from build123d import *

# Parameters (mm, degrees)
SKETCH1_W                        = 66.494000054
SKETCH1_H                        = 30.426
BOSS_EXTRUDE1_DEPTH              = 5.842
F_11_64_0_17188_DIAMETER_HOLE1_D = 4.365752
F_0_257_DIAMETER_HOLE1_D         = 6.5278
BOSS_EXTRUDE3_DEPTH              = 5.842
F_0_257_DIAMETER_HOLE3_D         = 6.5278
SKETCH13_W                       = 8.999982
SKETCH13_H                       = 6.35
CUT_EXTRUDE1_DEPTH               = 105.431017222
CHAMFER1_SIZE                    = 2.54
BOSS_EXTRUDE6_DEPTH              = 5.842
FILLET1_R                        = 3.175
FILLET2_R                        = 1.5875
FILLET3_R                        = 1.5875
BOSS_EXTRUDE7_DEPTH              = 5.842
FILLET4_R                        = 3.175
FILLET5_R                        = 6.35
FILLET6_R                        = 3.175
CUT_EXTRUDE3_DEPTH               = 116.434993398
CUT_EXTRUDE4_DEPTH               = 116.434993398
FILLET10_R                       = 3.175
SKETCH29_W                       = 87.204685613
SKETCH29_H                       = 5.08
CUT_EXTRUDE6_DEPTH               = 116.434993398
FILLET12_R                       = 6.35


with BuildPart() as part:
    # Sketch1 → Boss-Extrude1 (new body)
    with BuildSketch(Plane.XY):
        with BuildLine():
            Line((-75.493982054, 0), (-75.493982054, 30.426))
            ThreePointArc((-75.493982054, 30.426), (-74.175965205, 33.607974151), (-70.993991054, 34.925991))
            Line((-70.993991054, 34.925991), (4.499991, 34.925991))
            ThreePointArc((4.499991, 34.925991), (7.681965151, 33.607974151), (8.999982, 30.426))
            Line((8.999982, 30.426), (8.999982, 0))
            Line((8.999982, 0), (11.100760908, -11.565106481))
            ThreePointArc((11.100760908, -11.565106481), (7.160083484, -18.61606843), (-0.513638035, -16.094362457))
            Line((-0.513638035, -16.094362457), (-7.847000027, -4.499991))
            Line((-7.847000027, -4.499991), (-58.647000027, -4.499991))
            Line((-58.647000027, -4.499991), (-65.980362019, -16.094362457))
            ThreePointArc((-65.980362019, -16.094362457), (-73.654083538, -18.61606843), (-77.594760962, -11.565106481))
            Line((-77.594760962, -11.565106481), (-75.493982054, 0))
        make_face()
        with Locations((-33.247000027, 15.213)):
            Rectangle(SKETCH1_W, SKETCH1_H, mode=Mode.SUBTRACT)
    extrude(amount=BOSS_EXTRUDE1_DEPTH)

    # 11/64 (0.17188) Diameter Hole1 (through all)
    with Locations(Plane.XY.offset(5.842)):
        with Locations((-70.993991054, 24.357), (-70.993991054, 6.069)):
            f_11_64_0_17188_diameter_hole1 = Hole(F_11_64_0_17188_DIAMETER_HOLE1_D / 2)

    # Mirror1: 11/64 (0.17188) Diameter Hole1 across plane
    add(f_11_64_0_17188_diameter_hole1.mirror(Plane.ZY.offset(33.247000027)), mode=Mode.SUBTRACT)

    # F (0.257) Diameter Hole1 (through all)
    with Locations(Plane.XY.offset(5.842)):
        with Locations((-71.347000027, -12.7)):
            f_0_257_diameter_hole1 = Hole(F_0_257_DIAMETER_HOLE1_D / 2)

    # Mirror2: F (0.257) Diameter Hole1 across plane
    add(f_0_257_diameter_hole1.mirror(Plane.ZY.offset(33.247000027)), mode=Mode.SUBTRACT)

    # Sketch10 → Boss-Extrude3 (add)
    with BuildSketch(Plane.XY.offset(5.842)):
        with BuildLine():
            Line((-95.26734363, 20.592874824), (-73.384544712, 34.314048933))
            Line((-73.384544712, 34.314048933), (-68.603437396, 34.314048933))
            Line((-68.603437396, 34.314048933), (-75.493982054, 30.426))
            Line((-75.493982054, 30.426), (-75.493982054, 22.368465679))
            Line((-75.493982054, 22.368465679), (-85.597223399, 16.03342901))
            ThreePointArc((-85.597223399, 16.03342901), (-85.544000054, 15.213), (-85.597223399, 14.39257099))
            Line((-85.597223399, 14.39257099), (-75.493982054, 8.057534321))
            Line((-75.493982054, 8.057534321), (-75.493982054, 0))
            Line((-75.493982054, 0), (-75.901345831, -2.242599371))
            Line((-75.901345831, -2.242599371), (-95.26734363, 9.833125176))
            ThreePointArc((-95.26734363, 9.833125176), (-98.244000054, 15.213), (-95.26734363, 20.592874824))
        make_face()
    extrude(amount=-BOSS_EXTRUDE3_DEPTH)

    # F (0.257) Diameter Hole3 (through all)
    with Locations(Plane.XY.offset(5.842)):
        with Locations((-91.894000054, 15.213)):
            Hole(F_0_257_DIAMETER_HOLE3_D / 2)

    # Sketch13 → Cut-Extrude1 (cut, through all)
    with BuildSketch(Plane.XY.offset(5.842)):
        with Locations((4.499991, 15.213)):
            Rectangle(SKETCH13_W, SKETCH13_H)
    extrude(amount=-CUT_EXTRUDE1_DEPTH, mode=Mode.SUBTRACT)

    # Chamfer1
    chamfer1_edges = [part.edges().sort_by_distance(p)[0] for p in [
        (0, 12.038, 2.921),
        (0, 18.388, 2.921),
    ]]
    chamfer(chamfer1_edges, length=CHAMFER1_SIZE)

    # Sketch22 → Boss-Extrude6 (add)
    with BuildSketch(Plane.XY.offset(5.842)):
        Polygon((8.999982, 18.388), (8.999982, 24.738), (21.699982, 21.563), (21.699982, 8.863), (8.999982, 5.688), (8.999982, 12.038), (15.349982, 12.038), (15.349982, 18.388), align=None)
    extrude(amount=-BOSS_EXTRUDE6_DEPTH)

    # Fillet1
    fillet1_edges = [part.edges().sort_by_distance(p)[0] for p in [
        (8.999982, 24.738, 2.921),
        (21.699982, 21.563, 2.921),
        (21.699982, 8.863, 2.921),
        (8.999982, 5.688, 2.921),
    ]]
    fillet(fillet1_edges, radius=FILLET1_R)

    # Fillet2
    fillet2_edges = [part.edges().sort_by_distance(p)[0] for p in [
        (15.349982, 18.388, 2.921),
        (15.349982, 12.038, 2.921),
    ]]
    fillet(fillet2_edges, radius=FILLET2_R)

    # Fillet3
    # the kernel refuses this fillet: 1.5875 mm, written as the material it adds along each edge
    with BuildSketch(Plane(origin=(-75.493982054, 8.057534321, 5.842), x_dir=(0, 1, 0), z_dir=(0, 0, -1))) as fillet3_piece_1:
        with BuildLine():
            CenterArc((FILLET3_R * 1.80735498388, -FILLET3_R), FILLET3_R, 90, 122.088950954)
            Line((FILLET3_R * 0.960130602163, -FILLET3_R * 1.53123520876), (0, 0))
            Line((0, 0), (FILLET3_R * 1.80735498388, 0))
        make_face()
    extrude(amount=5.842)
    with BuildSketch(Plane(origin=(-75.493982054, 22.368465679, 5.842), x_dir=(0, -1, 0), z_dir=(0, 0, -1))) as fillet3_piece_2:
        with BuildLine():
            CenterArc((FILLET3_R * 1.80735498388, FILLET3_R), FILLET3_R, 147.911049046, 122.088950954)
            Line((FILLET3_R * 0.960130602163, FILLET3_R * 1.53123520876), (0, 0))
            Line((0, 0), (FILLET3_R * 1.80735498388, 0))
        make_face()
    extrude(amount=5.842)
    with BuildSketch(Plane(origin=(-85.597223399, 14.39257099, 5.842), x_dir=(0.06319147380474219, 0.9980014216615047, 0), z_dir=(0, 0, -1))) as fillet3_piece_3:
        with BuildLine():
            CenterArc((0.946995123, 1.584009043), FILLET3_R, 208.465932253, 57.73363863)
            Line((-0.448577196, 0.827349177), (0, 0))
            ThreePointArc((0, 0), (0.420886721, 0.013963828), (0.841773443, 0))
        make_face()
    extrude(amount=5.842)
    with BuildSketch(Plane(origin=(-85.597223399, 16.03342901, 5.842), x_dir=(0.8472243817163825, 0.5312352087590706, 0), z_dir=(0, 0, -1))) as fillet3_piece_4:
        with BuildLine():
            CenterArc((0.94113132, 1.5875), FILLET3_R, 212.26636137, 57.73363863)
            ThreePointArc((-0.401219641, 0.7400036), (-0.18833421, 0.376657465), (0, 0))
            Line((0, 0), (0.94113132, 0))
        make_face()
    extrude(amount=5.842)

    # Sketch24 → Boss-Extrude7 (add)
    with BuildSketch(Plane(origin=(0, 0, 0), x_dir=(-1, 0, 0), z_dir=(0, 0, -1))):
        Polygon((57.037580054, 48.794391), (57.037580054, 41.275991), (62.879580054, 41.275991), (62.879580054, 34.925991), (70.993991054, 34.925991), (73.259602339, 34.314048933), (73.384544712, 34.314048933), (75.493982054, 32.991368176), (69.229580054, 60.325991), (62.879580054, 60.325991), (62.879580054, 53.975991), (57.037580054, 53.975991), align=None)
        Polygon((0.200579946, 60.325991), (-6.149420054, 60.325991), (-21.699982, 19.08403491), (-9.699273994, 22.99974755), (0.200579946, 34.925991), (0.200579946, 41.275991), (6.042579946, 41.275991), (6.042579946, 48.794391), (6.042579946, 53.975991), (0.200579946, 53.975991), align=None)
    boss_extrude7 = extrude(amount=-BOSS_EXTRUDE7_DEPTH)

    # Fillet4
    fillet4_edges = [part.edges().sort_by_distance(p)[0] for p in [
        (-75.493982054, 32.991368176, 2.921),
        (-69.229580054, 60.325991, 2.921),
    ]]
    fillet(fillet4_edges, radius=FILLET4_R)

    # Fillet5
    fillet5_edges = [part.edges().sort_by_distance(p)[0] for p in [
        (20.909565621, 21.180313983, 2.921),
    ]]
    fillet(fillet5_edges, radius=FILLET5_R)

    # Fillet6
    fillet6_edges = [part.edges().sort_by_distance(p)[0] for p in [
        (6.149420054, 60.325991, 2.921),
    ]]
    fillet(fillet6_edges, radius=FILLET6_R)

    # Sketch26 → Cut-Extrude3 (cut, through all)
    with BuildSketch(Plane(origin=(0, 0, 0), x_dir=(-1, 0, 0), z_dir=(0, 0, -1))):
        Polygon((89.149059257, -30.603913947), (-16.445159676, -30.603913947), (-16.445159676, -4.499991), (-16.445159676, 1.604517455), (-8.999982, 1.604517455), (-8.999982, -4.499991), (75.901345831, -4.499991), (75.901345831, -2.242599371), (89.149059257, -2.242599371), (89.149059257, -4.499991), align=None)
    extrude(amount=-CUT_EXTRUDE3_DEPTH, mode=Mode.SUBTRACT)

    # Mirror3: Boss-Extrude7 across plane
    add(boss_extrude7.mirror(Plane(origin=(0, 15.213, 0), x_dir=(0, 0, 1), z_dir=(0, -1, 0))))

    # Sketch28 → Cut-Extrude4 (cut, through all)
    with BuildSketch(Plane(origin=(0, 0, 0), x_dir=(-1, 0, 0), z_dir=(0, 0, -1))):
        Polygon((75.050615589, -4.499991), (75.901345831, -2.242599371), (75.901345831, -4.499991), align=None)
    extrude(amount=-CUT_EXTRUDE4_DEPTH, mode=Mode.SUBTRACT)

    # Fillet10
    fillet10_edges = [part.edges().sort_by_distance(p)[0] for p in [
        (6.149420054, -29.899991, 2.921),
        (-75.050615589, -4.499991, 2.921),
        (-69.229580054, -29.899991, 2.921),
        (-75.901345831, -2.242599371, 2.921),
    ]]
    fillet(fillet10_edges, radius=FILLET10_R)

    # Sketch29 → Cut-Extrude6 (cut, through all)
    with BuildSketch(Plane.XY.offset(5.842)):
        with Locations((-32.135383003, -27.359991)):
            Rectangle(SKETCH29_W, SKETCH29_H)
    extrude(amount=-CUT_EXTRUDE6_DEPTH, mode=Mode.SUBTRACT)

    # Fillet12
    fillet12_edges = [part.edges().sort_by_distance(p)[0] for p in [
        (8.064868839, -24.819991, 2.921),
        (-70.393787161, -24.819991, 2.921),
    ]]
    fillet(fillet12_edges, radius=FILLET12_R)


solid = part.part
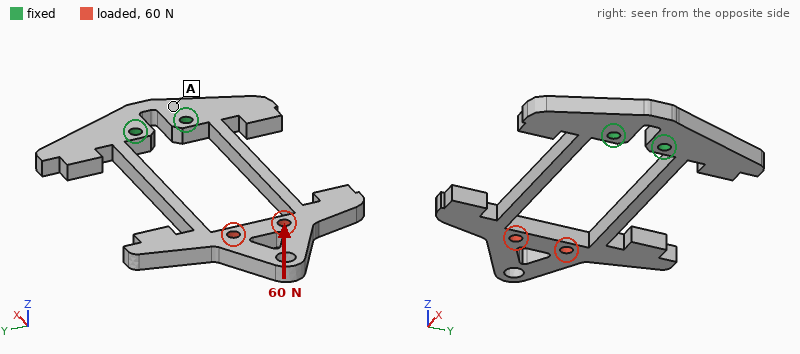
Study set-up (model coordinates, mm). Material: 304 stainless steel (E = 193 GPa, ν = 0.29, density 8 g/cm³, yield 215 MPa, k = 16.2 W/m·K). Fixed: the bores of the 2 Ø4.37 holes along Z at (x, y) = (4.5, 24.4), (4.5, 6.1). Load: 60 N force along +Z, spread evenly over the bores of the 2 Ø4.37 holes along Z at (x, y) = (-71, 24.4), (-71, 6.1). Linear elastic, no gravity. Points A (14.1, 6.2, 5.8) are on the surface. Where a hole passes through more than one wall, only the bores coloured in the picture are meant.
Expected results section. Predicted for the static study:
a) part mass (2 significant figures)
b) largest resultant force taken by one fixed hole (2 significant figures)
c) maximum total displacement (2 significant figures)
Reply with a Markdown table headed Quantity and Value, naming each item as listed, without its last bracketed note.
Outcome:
| Quantity | Value |
|---|---|
| part mass | 150 g |
| largest resultant force taken by one fixed hole | 30 N |
| maximum total displacement | 0.46 mm |
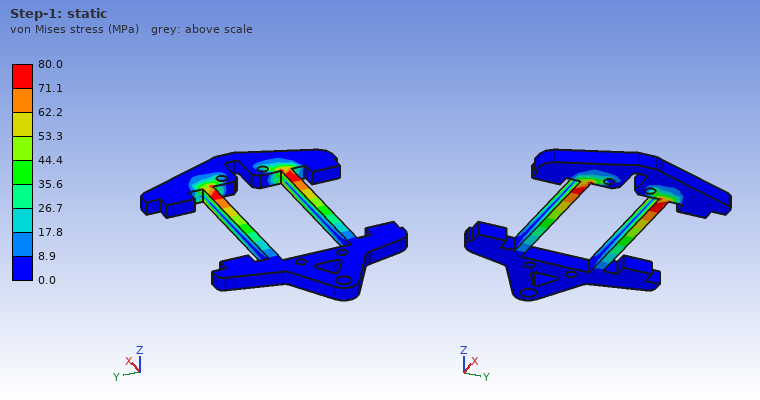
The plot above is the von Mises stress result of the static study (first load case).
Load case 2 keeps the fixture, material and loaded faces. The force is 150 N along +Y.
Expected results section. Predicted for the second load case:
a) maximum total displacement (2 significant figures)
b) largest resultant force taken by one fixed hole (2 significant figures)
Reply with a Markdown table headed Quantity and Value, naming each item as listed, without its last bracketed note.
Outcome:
| Quantity | Value |
|---|---|
| maximum total displacement | 0.25 mm |
| largest resultant force taken by one fixed hole | 310 N |
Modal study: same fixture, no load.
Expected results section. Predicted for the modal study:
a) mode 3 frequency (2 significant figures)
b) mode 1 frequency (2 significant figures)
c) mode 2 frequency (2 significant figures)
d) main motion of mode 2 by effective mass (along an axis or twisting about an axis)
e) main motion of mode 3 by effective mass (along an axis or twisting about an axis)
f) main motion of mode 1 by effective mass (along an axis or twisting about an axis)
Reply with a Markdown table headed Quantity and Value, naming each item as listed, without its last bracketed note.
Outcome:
| Quantity | Value |
|---|---|
| mode 3 frequency | 590 Hz |
| mode 1 frequency | 270 Hz |
| mode 2 frequency | 470 Hz |
| main motion of mode 2 by effective mass | along Y |
| main motion of mode 3 by effective mass | twisting about X |
| main motion of mode 1 by effective mass | along Z |
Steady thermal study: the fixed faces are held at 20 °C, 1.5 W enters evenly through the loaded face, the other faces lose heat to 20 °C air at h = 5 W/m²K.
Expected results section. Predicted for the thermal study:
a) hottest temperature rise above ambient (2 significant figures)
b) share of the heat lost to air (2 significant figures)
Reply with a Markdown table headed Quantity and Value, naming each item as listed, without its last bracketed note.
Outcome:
| Quantity | Value |
|---|---|
| hottest temperature rise above ambient | 47 K |
| share of the heat lost to air | 74 % |
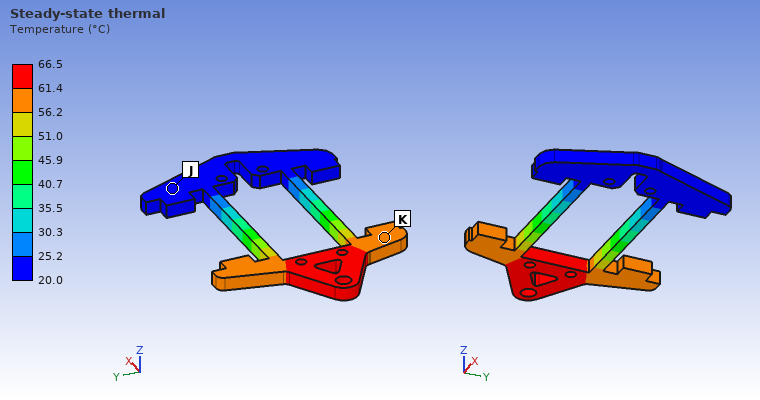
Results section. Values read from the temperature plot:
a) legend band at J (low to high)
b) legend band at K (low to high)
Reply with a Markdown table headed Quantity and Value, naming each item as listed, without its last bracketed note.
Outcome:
| Quantity | Value |
|---|---|
| legend band at J | 20.0 to 25.2 °C |
| legend band at K | 56.2 to 61.4 °C |
